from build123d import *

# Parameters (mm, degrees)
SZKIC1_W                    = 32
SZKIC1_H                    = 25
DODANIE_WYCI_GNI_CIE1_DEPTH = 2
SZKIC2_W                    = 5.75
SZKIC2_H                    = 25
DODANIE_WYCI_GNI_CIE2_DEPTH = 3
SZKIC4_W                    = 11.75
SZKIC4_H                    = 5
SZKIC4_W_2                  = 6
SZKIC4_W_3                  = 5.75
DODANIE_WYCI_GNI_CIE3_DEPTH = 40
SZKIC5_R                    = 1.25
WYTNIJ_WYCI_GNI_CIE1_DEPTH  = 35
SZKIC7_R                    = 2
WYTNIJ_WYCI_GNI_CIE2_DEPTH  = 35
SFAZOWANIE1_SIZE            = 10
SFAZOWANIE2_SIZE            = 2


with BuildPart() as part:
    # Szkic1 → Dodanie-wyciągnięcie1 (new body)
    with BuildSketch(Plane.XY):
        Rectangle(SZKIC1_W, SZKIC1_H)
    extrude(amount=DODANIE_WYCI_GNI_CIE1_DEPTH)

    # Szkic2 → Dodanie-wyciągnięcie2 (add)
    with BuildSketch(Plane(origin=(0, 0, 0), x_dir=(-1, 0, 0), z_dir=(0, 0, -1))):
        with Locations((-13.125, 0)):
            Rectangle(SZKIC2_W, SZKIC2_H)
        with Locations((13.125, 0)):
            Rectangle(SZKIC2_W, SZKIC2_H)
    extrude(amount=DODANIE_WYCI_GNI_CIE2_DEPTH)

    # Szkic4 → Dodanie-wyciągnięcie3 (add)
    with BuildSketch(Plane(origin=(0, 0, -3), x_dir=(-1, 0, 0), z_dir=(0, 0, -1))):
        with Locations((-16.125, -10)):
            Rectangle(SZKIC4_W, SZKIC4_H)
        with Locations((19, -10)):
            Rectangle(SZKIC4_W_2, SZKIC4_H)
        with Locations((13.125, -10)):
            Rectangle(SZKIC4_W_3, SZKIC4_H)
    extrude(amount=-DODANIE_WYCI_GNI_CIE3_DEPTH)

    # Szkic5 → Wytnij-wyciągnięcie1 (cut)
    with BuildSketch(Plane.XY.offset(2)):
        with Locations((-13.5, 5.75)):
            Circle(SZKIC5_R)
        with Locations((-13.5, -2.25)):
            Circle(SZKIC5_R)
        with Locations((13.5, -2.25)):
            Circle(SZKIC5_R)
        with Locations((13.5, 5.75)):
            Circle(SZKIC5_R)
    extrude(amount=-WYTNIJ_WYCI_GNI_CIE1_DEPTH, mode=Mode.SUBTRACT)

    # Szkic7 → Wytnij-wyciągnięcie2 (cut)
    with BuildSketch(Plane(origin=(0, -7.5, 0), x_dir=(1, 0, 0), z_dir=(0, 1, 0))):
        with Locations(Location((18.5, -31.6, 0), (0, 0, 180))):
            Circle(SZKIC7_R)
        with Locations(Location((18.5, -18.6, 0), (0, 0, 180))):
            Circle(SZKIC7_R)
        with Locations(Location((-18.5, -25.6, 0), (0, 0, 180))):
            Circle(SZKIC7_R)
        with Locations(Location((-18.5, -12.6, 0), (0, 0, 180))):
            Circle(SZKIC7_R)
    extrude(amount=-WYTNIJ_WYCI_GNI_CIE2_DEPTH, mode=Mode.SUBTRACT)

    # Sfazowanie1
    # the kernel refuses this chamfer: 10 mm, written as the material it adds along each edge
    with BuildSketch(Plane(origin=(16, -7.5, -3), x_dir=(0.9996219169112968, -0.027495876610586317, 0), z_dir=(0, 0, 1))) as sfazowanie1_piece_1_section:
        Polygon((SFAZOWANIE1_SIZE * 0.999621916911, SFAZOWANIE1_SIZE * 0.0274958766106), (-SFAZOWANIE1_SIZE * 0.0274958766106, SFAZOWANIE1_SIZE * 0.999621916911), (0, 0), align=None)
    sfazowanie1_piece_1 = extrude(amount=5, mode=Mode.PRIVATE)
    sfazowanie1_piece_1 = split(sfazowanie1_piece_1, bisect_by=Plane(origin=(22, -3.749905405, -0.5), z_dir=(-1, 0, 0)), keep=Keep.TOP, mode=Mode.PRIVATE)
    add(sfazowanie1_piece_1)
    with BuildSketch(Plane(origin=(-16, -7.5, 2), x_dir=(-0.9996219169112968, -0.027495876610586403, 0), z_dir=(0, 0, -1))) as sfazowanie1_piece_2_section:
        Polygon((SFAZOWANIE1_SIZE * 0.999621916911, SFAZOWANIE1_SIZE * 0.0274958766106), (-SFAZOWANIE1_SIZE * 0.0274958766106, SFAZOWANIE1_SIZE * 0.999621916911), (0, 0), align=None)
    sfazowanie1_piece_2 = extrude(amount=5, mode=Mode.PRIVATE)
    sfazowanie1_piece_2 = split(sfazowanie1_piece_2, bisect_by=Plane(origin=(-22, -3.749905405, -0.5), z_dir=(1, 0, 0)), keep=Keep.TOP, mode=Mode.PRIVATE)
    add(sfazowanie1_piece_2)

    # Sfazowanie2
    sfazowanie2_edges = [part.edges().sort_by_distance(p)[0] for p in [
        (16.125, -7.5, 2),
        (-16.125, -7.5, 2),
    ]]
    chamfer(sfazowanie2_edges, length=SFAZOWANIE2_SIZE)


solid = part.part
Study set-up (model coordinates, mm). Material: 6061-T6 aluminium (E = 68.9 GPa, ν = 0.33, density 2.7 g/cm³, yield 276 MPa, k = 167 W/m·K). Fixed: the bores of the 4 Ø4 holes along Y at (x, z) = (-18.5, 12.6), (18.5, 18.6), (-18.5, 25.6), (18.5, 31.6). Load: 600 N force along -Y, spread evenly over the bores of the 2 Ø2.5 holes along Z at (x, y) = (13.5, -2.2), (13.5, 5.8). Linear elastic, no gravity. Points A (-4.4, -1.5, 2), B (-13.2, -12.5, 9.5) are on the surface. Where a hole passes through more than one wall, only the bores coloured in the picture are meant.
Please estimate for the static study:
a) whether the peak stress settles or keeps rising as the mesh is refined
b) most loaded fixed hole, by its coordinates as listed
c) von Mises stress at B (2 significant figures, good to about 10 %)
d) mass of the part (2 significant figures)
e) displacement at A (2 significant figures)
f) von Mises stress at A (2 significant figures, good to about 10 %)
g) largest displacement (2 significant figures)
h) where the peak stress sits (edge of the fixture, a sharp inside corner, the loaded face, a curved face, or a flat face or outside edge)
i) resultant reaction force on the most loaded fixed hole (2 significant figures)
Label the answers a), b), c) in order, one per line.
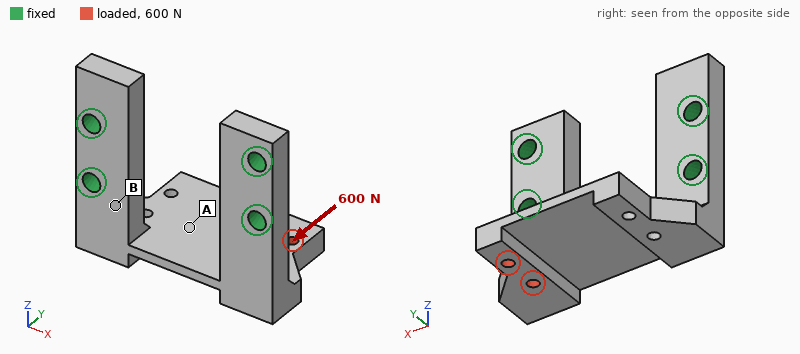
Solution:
a) keeps rising
b) (18.5, 18.6)
c) 43 MPa
d) 19 g
e) 0.057 mm
f) 13 MPa
g) 0.22 mm
h) edge of the fixture
i) 540 N
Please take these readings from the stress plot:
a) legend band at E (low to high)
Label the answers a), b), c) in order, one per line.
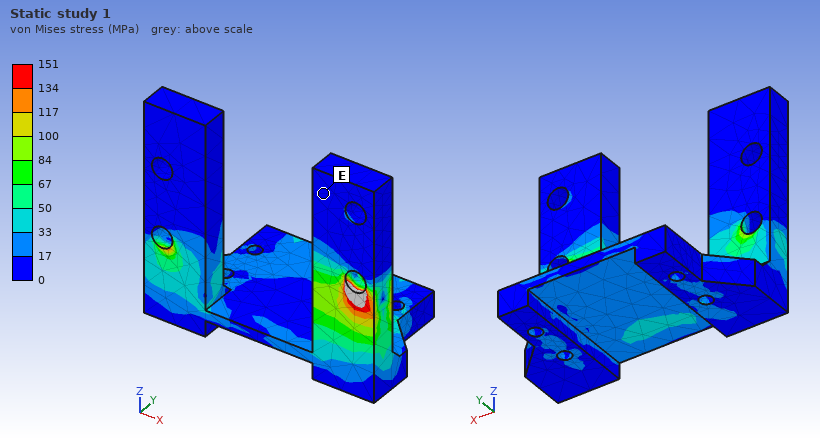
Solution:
a) 0 to 17 MPa
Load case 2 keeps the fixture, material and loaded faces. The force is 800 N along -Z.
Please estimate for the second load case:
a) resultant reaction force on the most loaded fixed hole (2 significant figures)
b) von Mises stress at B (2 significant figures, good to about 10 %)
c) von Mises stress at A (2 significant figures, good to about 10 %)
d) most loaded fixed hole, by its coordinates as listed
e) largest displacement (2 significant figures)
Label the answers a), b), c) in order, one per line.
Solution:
a) 640 N
b) 50 MPa
c) 49 MPa
d) (18.5, 18.6)
e) 0.41 mm
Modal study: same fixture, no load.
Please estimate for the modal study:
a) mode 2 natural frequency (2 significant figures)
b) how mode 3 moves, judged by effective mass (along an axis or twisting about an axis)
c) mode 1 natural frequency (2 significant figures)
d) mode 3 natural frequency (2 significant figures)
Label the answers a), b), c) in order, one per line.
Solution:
a) 6300 Hz
b) along Y
c) 3900 Hz
d) 9500 Hz
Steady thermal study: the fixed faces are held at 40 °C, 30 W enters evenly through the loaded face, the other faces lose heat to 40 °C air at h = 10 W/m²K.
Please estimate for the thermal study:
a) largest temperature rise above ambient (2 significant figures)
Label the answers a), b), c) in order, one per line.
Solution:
a) 62 K
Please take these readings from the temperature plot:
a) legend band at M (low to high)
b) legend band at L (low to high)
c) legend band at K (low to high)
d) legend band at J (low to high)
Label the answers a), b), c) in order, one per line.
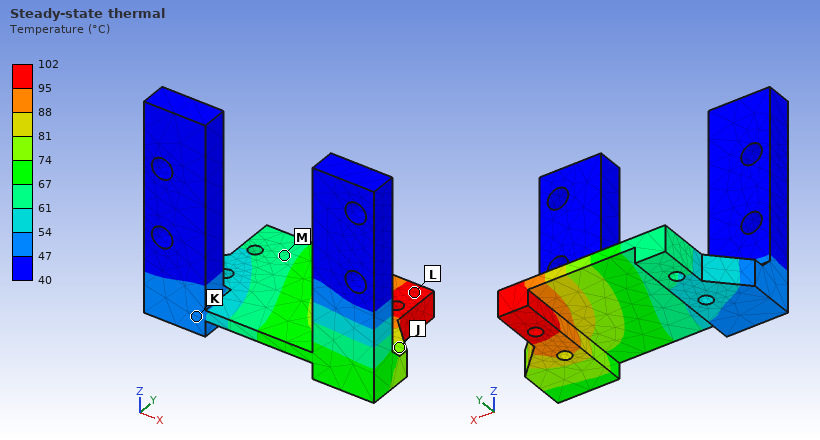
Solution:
a) 61 to 67 °C
b) 95 to 102 °C
c) 47 to 54 °C
d) 74 to 81 °C
